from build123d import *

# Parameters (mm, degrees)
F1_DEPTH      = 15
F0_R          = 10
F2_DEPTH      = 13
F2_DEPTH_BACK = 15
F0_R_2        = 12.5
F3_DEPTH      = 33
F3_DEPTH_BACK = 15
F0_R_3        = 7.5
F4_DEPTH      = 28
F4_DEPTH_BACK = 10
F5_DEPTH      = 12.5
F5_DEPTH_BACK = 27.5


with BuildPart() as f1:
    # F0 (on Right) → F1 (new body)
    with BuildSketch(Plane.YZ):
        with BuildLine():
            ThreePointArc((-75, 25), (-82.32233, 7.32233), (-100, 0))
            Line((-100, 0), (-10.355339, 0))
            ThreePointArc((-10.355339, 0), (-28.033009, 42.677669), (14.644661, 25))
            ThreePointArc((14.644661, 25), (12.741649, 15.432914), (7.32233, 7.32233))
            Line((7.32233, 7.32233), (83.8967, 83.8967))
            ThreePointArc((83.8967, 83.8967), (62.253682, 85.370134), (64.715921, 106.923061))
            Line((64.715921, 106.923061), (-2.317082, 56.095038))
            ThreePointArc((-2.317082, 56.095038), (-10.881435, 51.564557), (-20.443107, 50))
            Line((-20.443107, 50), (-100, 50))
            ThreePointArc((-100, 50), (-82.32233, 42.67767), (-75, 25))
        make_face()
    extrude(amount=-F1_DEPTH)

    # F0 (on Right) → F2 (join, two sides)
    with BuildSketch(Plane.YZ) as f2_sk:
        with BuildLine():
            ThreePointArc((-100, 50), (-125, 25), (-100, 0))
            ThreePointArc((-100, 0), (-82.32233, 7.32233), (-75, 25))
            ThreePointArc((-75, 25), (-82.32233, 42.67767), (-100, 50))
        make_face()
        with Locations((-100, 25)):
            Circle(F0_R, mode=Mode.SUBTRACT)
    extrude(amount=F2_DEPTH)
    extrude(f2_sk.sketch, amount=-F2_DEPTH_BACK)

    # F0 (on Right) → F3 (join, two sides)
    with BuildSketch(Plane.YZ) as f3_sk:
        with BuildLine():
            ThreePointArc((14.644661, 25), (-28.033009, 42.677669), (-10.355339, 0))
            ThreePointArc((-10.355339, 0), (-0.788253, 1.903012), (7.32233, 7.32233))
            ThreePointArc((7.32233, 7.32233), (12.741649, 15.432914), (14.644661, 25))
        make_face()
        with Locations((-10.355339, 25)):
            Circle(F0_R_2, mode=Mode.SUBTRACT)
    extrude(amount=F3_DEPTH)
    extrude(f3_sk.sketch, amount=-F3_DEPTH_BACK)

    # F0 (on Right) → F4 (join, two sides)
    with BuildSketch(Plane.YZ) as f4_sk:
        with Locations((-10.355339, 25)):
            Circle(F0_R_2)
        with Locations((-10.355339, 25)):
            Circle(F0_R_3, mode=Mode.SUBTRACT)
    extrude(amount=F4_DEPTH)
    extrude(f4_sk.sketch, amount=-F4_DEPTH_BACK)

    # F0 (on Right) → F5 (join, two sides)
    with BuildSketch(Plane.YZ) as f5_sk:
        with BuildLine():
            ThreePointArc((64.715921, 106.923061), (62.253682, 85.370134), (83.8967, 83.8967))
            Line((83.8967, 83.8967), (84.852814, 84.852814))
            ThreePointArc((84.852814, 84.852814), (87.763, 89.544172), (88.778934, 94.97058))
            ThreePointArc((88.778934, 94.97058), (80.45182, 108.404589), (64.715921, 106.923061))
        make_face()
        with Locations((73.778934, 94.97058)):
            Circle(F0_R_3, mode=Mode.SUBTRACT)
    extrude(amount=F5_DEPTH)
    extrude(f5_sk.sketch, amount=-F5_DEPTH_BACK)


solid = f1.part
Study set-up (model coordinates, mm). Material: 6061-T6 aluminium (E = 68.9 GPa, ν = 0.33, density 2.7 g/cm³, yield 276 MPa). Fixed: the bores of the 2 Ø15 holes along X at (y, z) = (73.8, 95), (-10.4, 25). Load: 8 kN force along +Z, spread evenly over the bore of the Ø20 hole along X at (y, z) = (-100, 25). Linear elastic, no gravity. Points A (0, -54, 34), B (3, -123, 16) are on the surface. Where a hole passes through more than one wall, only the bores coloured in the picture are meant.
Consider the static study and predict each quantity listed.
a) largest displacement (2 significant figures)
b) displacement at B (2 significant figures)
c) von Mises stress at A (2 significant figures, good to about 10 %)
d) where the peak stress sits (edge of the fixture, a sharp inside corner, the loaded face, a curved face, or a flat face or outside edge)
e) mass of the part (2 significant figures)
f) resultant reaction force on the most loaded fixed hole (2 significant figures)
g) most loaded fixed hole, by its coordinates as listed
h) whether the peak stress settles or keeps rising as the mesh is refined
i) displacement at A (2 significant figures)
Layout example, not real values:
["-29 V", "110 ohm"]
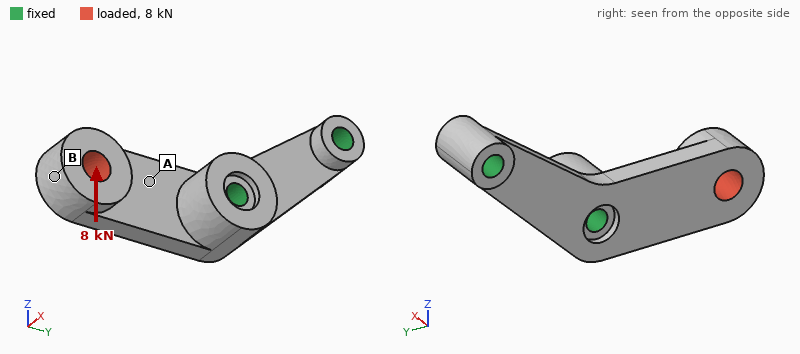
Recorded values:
["0.40 mm", "0.38 mm", "54 MPa", "edge of the fixture", "620 g", "9.1 kN", "(-10.4, 25)", "keeps rising", "0.10 mm"]
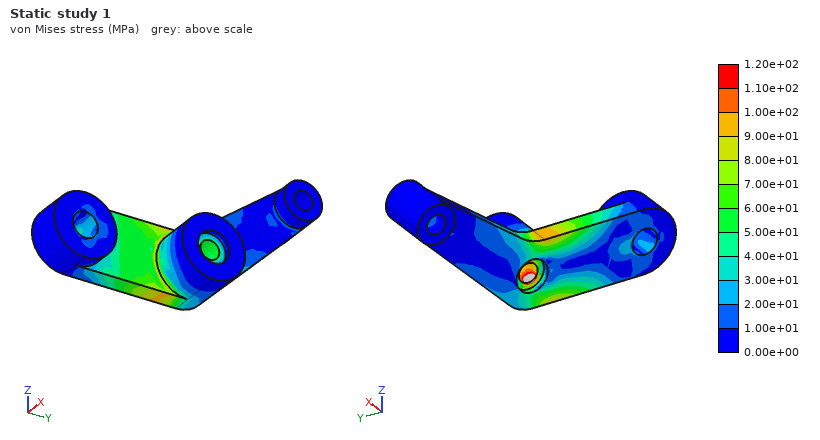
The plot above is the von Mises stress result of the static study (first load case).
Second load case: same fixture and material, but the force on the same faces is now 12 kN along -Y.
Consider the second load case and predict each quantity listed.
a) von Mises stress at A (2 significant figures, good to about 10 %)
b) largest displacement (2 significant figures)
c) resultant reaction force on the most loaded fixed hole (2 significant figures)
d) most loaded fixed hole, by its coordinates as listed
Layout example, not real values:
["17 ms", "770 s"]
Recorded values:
["56 MPa", "0.32 mm", "12 kN", "(-10.4, 25)"]
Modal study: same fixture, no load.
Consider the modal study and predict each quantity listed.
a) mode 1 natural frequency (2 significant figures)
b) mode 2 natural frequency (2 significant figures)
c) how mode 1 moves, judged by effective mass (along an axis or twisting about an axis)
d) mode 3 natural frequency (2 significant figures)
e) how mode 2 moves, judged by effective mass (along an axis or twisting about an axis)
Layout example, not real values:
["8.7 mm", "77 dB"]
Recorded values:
["1100 Hz", "2200 Hz", "along X", "3800 Hz", "along Z"]
